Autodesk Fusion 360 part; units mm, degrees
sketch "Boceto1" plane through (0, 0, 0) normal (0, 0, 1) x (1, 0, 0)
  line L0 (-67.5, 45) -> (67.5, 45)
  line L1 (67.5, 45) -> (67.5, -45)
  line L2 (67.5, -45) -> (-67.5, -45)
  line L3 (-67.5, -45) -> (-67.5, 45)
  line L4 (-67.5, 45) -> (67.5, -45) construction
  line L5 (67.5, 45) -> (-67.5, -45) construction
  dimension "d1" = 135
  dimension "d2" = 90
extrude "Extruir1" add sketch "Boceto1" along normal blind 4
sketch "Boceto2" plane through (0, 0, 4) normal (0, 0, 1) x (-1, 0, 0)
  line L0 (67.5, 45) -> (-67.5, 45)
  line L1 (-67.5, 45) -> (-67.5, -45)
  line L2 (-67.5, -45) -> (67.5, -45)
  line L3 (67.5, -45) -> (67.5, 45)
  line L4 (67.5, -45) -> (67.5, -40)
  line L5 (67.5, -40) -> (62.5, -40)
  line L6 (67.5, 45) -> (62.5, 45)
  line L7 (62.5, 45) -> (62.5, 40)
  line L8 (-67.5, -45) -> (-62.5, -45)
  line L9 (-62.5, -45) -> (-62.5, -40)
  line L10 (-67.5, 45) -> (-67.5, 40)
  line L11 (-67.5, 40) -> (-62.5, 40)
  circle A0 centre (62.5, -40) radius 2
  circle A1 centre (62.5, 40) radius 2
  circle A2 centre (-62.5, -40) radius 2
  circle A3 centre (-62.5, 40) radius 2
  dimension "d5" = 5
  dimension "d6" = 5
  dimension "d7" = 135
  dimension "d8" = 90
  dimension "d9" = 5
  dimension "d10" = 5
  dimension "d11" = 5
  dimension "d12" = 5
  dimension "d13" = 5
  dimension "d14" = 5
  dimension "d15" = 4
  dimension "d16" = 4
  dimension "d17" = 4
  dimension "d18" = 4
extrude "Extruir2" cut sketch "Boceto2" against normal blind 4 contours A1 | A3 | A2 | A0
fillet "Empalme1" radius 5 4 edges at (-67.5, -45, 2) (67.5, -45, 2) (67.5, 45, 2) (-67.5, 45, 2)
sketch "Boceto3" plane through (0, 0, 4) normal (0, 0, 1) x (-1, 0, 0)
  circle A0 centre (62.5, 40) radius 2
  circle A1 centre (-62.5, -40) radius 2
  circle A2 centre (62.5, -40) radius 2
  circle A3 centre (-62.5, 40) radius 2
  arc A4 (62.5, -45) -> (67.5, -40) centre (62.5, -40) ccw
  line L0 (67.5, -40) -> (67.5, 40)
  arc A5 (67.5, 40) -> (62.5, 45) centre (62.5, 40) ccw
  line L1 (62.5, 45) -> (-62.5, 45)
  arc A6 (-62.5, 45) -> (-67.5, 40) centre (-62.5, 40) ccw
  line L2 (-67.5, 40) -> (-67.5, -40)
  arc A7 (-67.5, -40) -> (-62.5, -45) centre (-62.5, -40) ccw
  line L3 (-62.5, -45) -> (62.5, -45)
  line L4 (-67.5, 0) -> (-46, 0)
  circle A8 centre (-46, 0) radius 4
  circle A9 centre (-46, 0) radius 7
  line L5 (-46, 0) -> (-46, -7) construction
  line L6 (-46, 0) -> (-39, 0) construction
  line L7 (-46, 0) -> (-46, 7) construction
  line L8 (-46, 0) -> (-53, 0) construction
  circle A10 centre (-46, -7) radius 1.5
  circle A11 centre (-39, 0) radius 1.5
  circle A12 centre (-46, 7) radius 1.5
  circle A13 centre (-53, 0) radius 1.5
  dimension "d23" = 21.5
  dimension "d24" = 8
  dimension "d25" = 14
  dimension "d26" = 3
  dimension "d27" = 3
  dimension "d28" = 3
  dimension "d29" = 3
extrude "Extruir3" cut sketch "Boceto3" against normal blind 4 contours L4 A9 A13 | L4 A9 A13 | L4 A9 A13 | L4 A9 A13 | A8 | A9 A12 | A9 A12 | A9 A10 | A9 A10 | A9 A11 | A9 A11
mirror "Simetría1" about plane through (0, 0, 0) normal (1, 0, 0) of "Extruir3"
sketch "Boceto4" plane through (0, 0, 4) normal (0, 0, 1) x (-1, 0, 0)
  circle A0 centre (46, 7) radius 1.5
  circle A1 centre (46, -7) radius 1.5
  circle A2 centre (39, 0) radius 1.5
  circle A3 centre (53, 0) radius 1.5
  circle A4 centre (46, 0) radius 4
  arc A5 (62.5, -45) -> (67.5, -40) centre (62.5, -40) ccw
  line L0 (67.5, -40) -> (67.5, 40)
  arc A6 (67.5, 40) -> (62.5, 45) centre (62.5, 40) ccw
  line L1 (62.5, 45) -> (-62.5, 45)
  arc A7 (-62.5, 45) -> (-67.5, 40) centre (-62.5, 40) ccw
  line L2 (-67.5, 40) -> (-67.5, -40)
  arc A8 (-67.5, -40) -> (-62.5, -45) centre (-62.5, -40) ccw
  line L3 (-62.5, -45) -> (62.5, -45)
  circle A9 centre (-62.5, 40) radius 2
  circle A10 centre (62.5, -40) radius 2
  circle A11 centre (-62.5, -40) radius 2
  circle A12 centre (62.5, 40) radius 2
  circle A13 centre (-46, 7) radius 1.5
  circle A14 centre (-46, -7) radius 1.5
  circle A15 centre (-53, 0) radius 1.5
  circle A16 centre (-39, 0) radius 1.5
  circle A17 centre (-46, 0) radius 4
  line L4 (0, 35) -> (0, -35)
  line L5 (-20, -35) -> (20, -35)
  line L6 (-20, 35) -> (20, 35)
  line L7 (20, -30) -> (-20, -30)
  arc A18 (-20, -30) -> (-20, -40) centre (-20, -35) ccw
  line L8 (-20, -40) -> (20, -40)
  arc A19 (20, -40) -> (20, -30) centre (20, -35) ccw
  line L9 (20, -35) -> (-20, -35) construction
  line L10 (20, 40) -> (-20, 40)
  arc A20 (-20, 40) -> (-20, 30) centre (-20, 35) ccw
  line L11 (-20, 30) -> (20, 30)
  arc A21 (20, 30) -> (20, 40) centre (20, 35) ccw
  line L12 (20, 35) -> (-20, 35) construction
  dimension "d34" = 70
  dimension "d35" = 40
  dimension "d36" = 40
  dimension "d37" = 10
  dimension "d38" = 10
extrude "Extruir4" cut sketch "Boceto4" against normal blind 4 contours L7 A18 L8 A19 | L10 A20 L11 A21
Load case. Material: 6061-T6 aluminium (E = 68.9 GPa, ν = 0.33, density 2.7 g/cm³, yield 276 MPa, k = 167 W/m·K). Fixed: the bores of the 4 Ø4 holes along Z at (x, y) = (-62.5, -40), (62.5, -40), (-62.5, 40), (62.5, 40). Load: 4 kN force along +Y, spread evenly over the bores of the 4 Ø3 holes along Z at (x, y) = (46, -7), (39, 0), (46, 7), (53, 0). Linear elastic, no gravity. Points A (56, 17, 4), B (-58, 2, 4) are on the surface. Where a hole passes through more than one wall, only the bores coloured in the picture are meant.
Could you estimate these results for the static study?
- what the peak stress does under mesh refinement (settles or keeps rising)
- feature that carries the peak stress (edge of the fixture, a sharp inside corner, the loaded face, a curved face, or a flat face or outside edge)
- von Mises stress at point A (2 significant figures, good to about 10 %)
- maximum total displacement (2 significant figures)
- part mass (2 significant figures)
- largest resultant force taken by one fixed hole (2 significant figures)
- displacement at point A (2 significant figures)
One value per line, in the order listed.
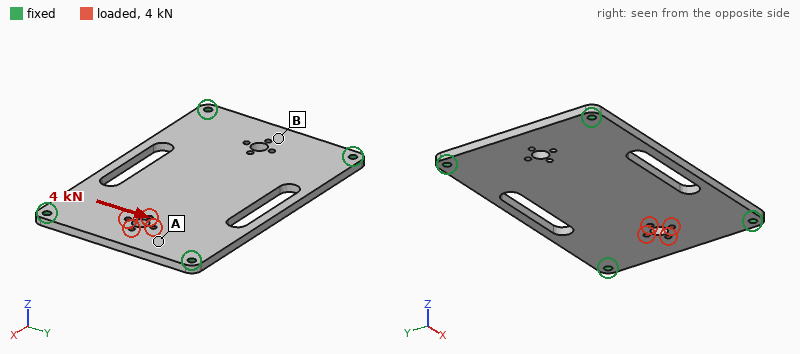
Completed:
keeps rising
edge of the fixture
21 MPa
19 µm
120 g
1.8 kN
10 µm
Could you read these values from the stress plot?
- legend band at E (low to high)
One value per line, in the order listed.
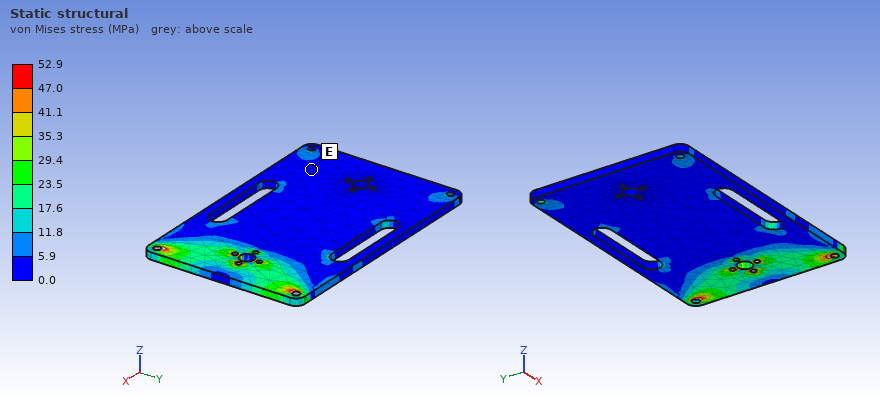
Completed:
0.0 to 5.9 MPa
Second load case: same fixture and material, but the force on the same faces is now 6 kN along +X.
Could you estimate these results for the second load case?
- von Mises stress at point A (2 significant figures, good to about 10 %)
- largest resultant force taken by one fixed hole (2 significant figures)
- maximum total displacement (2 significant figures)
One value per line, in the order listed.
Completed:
20 MPa
2.1 kN
37 µm
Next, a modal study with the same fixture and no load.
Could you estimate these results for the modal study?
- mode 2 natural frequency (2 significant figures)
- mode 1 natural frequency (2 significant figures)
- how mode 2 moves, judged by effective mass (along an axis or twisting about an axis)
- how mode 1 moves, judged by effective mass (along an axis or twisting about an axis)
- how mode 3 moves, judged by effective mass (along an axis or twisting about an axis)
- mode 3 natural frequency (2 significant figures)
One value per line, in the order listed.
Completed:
1900 Hz
1000 Hz
twisting about X
along Z
twisting about Y
2500 Hz
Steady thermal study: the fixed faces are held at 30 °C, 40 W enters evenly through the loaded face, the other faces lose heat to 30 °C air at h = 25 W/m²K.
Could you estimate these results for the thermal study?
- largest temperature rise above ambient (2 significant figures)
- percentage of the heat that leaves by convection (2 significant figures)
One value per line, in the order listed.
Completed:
34 K
18 %
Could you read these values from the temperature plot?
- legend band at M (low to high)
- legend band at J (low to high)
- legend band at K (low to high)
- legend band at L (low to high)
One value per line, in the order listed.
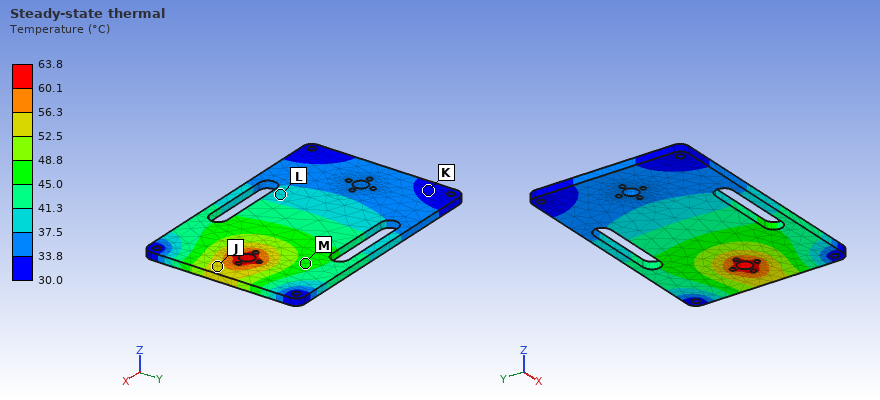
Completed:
45.0 to 48.8 °C
52.5 to 56.3 °C
30.0 to 33.8 °C
37.5 to 41.3 °C
